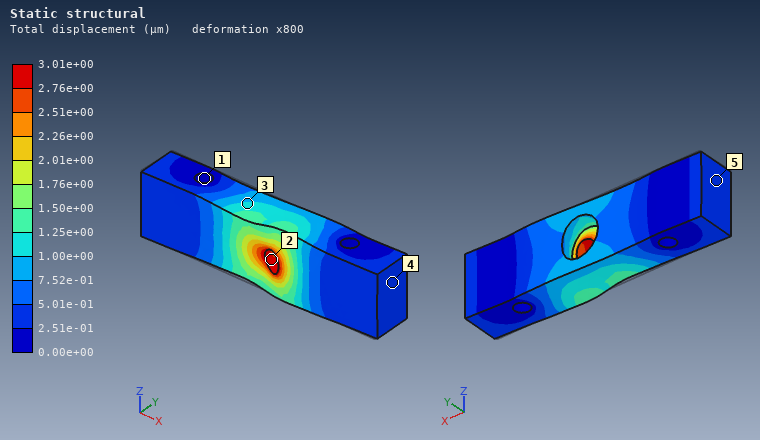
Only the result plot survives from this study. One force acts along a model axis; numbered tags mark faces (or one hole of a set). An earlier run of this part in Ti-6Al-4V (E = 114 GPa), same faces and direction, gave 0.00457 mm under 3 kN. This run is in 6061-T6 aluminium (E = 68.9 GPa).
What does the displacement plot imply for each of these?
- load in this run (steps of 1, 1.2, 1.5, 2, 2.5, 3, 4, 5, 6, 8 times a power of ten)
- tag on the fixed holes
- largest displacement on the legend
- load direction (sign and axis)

1.2 kN
1
3.01e+00 µm
+X
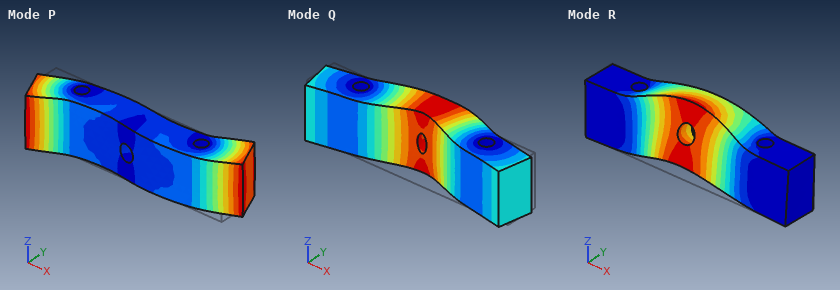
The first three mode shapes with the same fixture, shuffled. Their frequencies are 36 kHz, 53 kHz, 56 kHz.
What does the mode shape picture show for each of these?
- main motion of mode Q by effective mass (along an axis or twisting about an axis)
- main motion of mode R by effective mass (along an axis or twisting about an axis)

along Y
along Z
